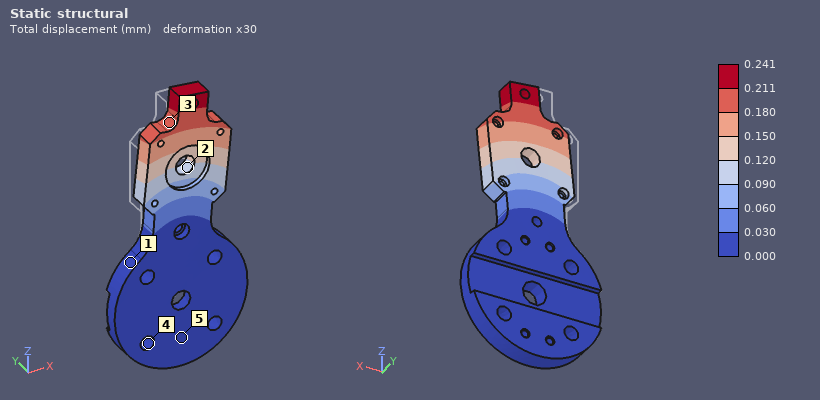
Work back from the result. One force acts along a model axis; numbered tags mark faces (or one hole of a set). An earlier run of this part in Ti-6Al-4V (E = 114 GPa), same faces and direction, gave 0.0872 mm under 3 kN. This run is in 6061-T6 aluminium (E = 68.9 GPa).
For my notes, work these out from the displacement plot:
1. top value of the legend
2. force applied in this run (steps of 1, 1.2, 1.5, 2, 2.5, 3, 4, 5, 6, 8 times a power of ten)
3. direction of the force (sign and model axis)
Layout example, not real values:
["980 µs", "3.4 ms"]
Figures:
["0.241 mm", "5 kN", "+X"]
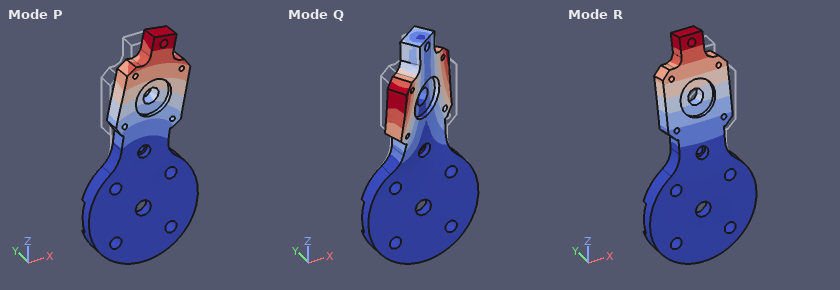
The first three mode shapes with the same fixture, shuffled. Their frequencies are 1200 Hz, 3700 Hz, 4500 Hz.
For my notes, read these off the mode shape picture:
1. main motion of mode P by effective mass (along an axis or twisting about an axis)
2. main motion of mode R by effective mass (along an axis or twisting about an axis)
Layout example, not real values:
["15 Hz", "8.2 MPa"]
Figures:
["along X", "along Y"]
